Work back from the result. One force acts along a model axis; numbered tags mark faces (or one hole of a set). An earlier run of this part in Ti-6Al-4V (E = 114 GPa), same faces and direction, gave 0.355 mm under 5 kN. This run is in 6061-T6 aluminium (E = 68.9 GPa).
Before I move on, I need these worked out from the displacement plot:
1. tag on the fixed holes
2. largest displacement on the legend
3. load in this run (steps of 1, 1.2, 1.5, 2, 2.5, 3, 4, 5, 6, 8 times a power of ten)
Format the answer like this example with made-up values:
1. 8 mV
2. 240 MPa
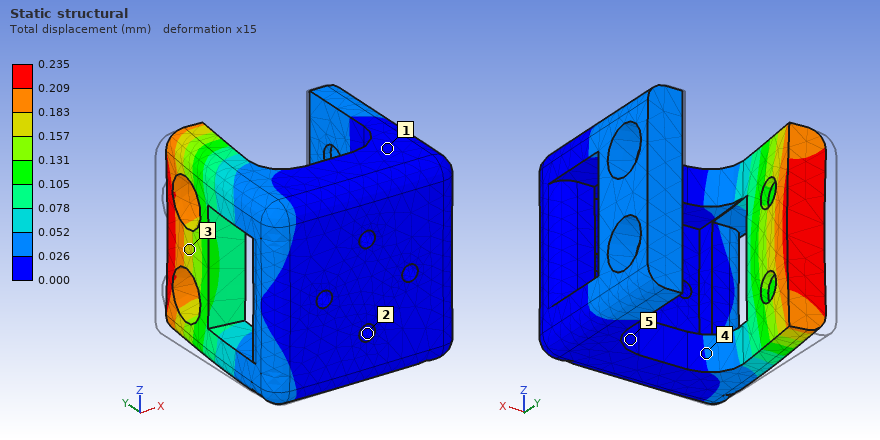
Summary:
1. 2
2. 0.235 mm
3. 2 kN
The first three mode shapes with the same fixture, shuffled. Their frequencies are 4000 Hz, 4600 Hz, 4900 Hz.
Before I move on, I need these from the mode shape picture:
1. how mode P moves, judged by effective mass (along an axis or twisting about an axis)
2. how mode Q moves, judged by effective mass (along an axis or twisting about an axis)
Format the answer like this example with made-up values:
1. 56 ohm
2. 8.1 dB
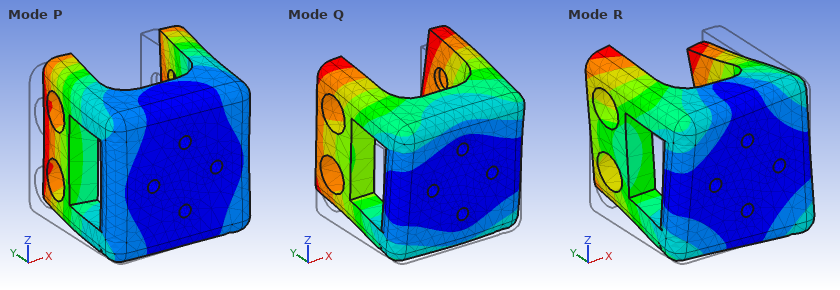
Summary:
1. along X
2. along Z
